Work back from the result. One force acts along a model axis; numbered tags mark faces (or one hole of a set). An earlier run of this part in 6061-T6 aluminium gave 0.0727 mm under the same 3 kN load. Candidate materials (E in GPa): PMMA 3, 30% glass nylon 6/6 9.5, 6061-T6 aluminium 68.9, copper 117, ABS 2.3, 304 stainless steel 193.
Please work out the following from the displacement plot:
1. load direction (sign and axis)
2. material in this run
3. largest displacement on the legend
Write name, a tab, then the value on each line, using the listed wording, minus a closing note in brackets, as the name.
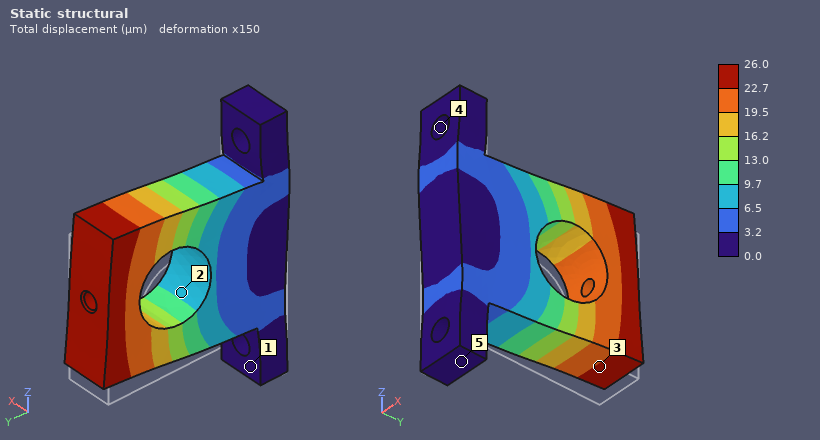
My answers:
load direction	+Z
material in this run	304 stainless steel
largest displacement on the legend	26.0 µm
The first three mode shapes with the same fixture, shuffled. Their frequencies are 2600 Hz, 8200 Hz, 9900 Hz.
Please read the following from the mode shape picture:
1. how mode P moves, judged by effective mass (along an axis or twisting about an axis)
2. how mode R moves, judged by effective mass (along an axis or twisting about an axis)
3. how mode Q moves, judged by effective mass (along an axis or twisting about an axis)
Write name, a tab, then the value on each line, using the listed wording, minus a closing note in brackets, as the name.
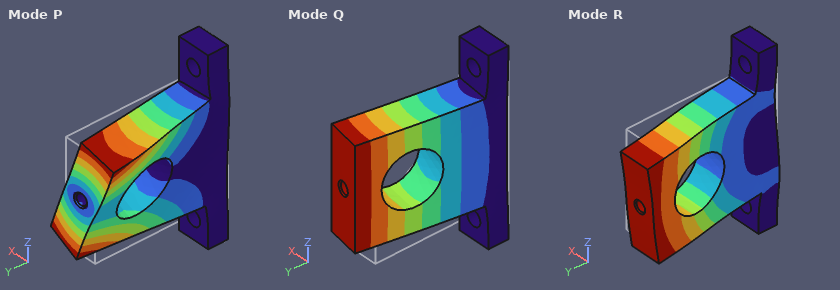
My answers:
how mode P moves, judged by effective mass	twisting about Y
how mode R moves, judged by effective mass	along Z
how mode Q moves, judged by effective mass	along X
